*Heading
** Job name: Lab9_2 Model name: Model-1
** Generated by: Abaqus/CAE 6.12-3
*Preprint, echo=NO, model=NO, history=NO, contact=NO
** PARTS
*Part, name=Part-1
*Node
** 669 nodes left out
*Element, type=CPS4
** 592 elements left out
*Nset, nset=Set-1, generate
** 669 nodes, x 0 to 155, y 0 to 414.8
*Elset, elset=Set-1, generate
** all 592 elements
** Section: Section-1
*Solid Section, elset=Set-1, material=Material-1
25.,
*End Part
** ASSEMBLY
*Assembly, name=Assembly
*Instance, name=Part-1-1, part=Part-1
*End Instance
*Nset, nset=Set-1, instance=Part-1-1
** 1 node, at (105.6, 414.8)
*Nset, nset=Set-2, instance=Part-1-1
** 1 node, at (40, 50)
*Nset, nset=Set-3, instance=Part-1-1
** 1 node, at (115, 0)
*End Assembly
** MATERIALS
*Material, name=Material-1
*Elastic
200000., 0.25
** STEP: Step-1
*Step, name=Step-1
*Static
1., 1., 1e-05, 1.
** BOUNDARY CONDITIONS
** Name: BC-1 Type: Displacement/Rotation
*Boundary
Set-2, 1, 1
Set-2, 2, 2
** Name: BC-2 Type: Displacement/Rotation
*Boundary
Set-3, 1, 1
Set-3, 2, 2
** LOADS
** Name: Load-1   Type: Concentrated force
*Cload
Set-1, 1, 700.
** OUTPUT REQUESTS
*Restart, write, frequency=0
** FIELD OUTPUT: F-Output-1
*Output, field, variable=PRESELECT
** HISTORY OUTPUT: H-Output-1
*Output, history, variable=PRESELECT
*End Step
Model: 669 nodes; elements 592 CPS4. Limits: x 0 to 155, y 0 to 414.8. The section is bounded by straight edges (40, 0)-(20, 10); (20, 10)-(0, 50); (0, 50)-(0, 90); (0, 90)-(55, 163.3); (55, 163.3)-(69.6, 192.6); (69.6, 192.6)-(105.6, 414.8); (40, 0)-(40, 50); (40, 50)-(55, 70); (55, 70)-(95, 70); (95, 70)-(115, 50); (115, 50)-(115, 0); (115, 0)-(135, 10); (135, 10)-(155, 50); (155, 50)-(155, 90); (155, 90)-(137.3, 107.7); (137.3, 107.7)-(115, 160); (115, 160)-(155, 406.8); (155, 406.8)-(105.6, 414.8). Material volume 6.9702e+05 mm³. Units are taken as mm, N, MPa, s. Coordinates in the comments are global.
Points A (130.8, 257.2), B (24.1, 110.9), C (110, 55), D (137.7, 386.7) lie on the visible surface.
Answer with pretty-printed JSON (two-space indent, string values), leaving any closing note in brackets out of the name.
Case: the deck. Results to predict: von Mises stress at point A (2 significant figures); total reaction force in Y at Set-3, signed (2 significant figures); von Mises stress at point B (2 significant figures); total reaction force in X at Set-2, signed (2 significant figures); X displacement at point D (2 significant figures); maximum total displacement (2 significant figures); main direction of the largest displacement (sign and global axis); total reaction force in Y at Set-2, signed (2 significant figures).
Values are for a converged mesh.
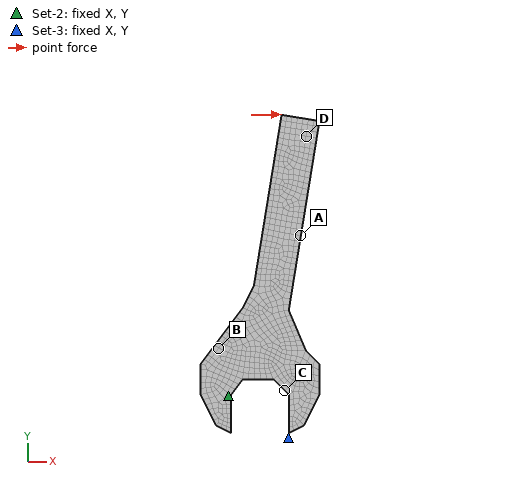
{
  "von Mises stress at point A": "10 MPa",
  "total reaction force in Y at Set-3, signed": "2800 N",
  "von Mises stress at point B": "1.3 MPa",
  "total reaction force in X at Set-2, signed": "-1700 N",
  "X displacement at point D": "0.11 mm",
  "maximum total displacement": "0.13 mm",
  "main direction of the largest displacement": "+X",
  "total reaction force in Y at Set-2, signed": "-2800 N"
}
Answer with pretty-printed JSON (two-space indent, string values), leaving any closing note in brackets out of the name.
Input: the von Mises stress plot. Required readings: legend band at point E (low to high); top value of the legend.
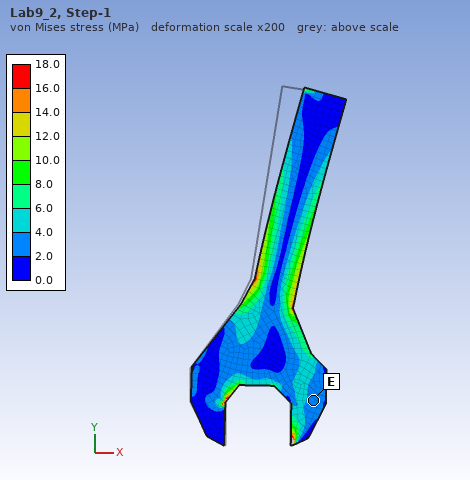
{
  "legend band at point E": "2.0 to 4.0 MPa",
  "top value of the legend": "18.0 MPa"
}
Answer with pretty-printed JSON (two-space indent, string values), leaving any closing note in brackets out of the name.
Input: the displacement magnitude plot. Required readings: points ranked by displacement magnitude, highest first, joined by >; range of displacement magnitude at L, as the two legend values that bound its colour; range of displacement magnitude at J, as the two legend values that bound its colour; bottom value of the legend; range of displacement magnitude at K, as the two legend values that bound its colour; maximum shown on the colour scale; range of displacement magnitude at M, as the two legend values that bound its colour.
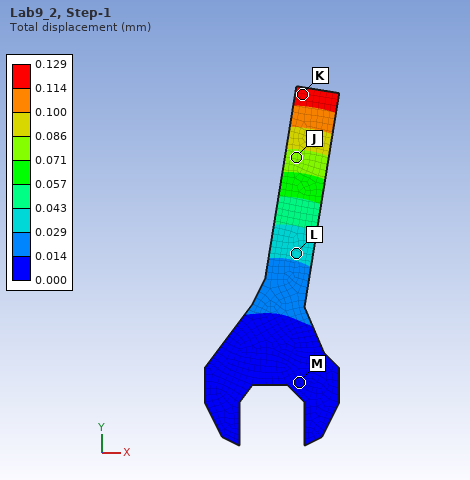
{
  "points ranked by displacement magnitude, highest first, joined by >": "K > J > L > M",
  "range of displacement magnitude at L, as the two legend values that bound its colour": "0.029 to 0.043 mm",
  "range of displacement magnitude at J, as the two legend values that bound its colour": "0.071 to 0.086 mm",
  "bottom value of the legend": "0.000 mm",
  "range of displacement magnitude at K, as the two legend values that bound its colour": "0.114 to 0.129 mm",
  "maximum shown on the colour scale": "0.129 mm",
  "range of displacement magnitude at M, as the two legend values that bound its colour": "0.000 to 0.014 mm"
}
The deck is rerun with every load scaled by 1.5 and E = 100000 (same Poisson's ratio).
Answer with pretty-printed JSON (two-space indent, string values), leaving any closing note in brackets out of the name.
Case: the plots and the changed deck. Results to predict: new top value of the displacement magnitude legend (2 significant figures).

{
  "new top value of the displacement magnitude legend": "0.39 mm"
}
